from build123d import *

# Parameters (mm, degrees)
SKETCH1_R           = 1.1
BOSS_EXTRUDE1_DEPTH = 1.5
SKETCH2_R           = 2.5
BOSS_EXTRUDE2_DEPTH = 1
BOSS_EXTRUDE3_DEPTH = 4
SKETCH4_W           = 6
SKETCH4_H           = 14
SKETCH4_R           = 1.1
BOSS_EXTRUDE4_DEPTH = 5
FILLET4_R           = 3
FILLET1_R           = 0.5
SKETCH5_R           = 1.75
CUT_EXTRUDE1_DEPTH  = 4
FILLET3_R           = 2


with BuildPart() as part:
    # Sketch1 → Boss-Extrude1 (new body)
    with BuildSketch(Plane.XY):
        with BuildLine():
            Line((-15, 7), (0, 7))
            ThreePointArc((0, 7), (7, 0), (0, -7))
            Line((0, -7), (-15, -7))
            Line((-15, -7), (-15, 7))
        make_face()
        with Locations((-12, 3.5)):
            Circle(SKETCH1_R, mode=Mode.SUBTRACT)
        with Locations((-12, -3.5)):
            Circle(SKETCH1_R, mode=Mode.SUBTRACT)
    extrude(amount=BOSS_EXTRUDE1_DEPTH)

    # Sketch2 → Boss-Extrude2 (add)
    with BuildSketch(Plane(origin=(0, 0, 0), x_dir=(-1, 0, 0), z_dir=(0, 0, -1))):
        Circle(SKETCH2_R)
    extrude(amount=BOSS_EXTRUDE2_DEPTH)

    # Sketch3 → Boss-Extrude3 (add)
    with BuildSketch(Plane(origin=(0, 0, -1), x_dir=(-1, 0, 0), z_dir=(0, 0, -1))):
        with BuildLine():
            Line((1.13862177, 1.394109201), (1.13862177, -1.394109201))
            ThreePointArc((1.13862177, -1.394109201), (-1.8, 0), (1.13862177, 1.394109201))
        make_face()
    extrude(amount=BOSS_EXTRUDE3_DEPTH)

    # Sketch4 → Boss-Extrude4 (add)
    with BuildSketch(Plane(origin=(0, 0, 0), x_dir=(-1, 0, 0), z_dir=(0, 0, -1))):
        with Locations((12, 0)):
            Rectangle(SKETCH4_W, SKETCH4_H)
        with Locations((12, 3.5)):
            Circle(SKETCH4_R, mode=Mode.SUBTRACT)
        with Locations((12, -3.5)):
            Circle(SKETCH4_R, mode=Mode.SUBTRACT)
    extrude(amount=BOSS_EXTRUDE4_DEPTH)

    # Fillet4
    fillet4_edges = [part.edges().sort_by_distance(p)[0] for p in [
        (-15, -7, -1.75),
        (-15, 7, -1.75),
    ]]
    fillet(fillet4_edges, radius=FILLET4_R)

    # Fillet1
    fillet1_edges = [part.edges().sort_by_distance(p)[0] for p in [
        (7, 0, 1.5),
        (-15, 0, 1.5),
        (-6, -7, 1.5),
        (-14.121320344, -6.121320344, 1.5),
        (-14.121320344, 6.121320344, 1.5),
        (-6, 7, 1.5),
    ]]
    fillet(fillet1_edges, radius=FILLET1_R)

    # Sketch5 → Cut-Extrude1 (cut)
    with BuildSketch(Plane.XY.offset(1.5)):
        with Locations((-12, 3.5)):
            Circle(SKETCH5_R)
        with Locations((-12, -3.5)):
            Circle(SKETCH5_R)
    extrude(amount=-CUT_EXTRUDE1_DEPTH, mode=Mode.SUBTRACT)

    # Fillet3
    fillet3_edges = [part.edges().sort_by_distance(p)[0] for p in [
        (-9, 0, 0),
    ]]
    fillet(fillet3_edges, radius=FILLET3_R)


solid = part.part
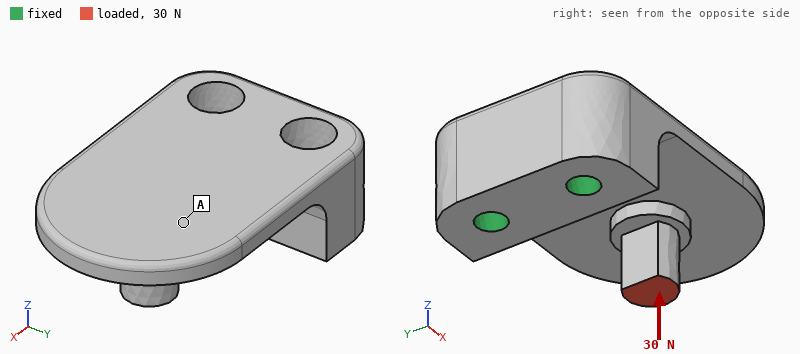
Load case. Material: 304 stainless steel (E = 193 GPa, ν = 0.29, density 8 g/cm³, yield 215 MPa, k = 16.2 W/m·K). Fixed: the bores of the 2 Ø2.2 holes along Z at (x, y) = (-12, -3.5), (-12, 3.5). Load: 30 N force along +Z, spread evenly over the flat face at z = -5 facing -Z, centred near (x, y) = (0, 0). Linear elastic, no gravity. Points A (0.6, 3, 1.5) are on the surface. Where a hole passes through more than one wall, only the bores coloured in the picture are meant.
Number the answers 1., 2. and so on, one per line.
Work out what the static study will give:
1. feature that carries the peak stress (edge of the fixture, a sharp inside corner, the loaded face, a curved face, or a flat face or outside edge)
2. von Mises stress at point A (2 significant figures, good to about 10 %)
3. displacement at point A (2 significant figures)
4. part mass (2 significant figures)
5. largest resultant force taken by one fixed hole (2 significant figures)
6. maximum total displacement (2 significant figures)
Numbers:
1. a curved face
2. 5.5 MPa
3. 12 µm
4. 6.3 g
5. 17 N
6. 22 µm
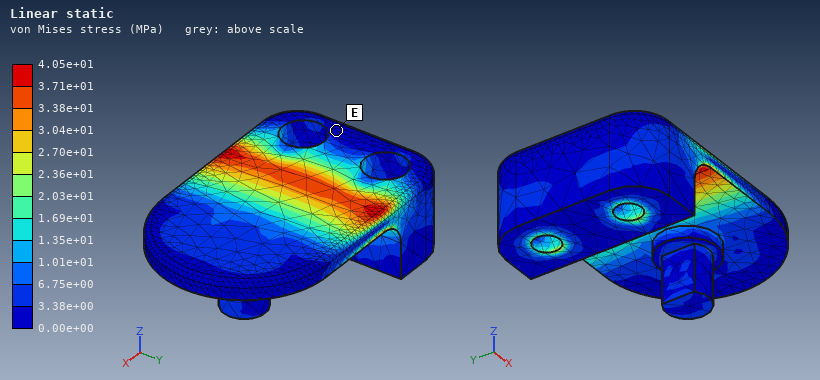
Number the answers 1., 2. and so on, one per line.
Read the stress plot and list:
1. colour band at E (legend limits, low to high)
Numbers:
1. 0.00e+00 to 3.38e+00 MPa
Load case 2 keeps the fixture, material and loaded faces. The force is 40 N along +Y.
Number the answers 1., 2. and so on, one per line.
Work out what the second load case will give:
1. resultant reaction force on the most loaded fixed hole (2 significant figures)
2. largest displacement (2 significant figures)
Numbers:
1. 51 N
2. 9.4 µm
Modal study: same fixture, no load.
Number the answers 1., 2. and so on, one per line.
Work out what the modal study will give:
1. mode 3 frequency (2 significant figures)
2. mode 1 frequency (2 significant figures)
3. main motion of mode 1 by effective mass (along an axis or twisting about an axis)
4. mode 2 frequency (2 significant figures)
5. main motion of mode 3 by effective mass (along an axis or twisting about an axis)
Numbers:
1. 20 kHz
2. 5000 Hz
3. along Z
4. 14 kHz
5. along Y
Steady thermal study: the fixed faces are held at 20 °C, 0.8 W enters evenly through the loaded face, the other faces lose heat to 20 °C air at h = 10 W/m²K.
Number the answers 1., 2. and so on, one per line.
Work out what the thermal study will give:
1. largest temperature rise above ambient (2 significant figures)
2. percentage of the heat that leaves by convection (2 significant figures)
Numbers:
1. 51 K
2. 14 %
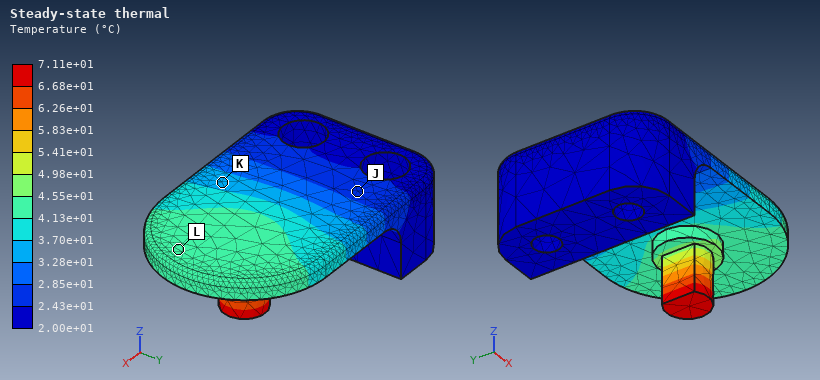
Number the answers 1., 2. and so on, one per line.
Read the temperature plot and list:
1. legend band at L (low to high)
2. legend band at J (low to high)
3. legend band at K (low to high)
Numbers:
1. 4.13e+01 to 4.55e+01 °C
2. 2.43e+01 to 2.85e+01 °C
3. 3.28e+01 to 3.70e+01 °C
